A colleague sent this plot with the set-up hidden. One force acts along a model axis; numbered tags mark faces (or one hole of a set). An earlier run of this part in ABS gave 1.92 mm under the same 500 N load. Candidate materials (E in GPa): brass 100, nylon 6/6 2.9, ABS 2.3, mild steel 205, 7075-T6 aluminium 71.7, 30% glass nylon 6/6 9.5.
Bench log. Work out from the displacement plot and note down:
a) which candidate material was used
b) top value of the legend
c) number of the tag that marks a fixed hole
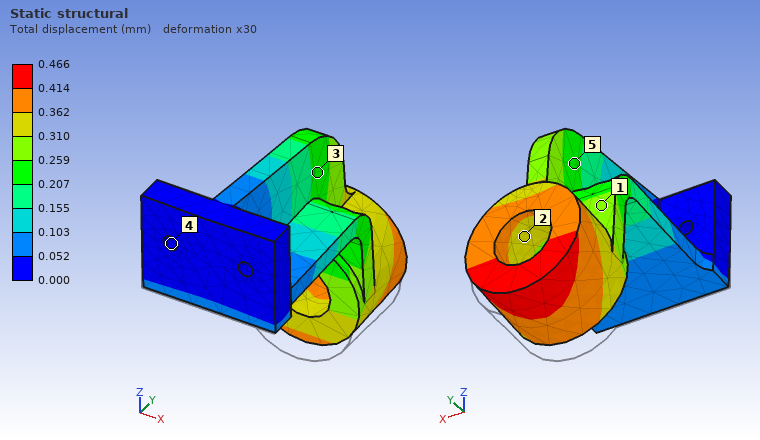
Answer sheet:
30% glass nylon 6/6
0.466 mm
4
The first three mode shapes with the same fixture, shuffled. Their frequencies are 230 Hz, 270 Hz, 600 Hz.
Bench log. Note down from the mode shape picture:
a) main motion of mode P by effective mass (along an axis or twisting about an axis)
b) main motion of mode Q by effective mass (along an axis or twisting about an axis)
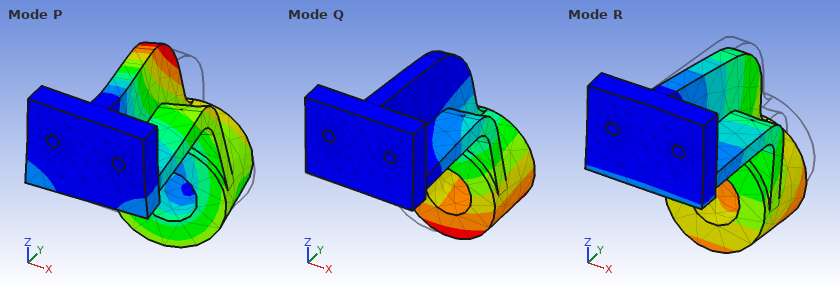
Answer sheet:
along X
along X
